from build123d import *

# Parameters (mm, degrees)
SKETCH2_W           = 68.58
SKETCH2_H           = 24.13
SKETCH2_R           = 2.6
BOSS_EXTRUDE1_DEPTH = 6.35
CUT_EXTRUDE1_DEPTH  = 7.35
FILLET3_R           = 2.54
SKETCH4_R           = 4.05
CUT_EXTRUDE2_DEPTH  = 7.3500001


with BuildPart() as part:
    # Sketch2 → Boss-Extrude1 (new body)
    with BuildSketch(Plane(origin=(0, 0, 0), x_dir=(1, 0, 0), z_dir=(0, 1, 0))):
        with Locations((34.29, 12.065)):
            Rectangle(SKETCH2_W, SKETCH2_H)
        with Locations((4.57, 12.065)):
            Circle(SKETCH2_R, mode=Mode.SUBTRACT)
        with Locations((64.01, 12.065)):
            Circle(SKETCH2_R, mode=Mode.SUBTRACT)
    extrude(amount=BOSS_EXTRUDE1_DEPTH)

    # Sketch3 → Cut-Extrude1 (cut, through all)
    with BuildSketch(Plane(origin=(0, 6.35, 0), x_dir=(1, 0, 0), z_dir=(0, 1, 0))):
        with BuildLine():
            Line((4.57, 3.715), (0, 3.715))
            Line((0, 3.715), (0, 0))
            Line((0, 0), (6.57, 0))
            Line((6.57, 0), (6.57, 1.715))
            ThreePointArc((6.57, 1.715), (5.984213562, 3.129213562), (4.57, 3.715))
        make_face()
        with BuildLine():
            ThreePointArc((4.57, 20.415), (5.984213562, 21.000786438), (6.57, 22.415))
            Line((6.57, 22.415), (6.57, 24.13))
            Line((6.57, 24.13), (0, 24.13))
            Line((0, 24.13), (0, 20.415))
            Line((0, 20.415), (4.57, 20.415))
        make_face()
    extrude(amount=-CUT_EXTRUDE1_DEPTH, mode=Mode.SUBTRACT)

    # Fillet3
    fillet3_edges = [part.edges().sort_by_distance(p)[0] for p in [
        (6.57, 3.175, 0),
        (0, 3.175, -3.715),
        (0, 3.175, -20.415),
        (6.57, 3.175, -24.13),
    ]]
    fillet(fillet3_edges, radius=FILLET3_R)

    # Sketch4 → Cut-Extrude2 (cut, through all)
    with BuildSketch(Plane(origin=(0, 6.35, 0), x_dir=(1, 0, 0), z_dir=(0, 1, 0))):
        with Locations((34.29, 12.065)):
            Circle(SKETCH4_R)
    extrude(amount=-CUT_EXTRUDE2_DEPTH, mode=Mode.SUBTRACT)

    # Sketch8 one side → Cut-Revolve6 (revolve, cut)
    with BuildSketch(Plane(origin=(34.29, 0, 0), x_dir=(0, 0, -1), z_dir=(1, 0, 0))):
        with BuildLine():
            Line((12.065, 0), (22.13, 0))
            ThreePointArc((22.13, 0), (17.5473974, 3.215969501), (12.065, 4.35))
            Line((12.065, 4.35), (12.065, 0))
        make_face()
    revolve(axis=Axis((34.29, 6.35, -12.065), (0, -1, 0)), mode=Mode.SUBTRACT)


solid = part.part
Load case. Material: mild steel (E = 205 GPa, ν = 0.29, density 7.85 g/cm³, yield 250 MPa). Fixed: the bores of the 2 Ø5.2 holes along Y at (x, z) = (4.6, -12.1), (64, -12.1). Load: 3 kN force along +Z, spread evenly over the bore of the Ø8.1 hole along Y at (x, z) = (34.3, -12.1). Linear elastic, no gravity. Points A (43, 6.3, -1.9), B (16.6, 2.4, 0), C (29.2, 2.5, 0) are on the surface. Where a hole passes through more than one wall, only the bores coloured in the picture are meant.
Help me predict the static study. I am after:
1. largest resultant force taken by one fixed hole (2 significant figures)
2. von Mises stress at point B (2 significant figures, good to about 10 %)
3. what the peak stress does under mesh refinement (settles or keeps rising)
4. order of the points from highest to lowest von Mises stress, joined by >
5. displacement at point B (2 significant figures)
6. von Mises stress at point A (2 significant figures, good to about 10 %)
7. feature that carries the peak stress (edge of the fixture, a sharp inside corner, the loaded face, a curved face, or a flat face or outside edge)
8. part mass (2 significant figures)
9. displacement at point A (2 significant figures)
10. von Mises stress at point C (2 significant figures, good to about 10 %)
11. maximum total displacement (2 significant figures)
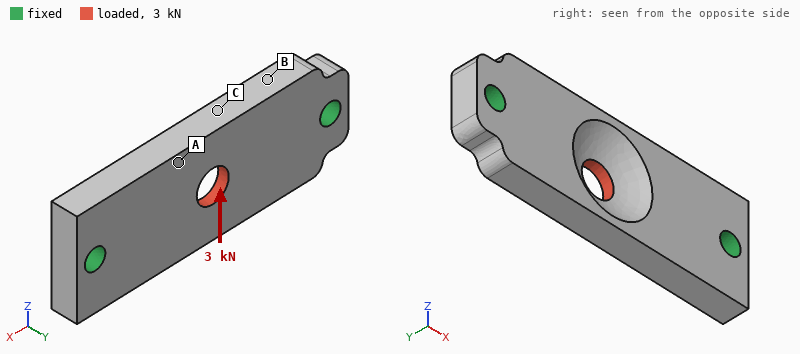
1.5 kN
16 MPa
keeps rising
C > A > B
6.4 µm
34 MPa
edge of the fixture
71 g
10 µm
56 MPa
13 µm
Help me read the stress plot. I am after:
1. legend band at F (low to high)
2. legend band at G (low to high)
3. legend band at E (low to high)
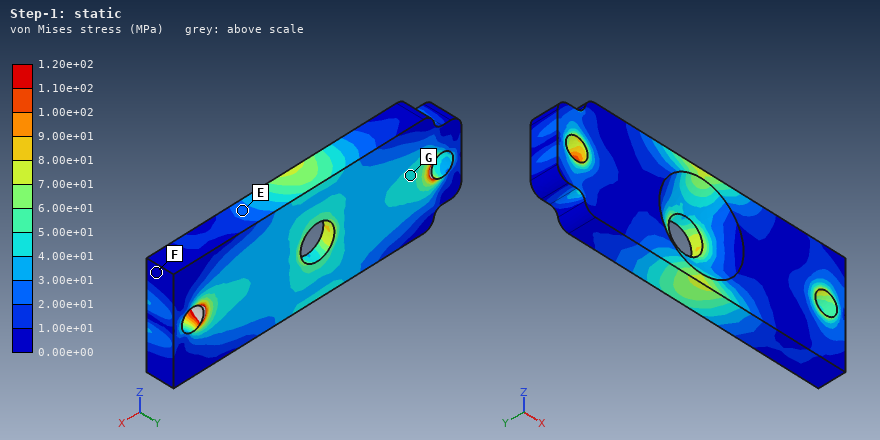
0.00e+00 to 1.00e+01 MPa
4.00e+01 to 5.00e+01 MPa
2.00e+01 to 3.00e+01 MPa
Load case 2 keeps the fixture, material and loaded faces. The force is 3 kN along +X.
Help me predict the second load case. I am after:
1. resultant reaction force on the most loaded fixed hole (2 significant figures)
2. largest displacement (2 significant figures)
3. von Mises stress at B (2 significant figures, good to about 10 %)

1.5 kN
2.9 µm
5.7 MPa
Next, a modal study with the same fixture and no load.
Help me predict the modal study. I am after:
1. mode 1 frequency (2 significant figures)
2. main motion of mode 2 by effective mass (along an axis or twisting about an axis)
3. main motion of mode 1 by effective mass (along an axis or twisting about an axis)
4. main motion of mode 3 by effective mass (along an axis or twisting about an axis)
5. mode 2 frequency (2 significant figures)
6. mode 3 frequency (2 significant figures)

8500 Hz
twisting about X
along Y
along Z
12 kHz
17 kHz
